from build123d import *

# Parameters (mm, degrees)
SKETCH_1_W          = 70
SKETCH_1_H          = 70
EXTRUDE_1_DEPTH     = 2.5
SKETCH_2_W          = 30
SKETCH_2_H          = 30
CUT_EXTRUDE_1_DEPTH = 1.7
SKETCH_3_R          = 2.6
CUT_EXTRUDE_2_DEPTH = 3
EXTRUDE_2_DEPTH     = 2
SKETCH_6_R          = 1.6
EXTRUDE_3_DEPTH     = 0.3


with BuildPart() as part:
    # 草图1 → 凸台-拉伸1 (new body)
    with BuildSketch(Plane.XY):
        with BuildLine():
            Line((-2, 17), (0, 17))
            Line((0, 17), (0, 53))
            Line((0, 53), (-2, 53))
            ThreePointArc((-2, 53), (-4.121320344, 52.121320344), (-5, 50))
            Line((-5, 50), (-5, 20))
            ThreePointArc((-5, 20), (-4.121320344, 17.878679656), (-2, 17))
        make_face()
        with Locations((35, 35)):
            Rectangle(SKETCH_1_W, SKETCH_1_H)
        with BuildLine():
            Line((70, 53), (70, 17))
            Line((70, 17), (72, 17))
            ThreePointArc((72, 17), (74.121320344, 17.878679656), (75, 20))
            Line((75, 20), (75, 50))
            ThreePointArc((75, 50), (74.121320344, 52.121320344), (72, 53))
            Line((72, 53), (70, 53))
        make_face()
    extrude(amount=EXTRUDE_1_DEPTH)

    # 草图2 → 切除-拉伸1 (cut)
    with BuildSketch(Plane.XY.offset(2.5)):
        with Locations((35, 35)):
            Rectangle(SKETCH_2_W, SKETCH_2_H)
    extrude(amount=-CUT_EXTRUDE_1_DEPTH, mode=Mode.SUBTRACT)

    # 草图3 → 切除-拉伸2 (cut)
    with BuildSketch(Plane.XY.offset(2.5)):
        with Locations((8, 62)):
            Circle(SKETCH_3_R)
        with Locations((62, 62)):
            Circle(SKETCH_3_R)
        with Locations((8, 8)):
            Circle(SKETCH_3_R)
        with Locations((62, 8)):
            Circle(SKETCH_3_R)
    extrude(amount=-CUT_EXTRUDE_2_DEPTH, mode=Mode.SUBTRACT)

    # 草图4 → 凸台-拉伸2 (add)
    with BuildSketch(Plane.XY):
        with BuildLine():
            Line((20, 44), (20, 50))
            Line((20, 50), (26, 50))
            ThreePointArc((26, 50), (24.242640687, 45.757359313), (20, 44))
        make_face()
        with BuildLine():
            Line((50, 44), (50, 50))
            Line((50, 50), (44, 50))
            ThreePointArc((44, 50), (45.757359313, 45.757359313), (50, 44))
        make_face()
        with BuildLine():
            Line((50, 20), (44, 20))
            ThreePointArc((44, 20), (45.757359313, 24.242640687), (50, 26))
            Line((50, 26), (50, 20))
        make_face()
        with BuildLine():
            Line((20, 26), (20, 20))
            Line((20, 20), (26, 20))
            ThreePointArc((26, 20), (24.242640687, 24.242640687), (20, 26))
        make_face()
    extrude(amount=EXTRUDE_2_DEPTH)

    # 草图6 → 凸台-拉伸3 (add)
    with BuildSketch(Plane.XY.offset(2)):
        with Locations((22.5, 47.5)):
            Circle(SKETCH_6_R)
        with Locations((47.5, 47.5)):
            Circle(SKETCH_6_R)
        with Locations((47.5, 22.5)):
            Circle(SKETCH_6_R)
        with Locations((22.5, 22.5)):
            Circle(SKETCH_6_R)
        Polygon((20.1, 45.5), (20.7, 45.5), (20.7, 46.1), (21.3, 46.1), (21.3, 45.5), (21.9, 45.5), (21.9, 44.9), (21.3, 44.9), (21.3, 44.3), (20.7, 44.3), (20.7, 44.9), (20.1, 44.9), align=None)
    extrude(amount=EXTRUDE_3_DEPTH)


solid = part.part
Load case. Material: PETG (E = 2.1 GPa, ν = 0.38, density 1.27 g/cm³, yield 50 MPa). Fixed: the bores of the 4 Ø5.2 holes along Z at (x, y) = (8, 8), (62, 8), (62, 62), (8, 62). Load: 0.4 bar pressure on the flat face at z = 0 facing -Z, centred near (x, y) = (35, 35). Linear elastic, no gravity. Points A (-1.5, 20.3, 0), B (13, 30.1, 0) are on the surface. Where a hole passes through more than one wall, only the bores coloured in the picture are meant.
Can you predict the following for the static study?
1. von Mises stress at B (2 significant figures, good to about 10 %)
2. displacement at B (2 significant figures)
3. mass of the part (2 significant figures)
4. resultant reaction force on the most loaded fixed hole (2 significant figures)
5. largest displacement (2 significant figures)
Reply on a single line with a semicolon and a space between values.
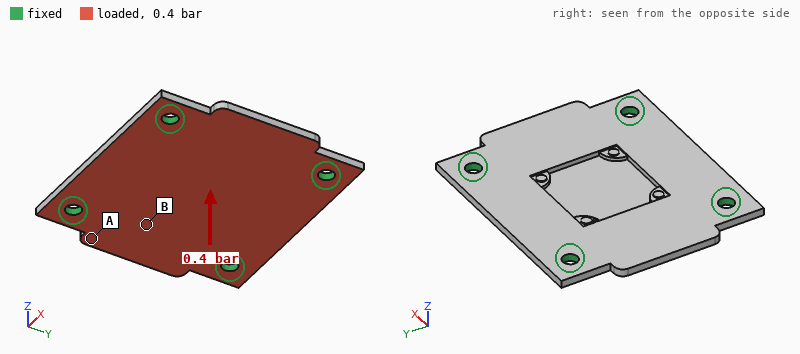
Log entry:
5.1 MPa; 0.47 mm; 15 g; 61 N; 1.2 mm
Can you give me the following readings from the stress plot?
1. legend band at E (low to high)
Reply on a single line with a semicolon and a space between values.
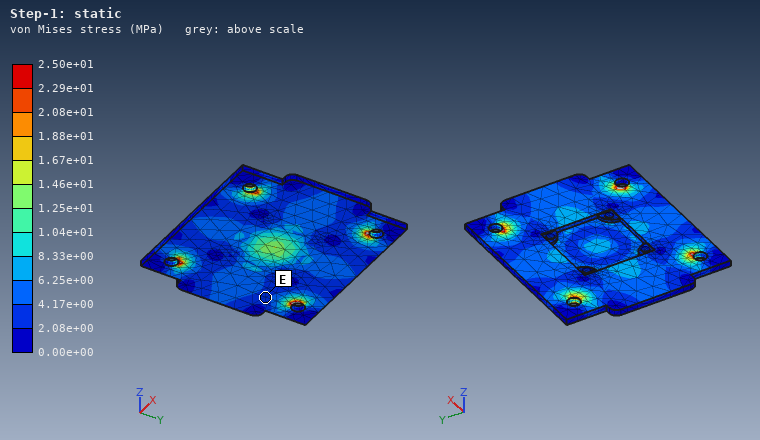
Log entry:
2.08e+00 to 4.17e+00 MPa
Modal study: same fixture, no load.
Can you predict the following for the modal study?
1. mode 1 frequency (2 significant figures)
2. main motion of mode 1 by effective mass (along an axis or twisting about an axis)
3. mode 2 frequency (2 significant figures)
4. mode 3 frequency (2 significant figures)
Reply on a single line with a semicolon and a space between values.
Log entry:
960 Hz; along Z; 1200 Hz; 1200 Hz
